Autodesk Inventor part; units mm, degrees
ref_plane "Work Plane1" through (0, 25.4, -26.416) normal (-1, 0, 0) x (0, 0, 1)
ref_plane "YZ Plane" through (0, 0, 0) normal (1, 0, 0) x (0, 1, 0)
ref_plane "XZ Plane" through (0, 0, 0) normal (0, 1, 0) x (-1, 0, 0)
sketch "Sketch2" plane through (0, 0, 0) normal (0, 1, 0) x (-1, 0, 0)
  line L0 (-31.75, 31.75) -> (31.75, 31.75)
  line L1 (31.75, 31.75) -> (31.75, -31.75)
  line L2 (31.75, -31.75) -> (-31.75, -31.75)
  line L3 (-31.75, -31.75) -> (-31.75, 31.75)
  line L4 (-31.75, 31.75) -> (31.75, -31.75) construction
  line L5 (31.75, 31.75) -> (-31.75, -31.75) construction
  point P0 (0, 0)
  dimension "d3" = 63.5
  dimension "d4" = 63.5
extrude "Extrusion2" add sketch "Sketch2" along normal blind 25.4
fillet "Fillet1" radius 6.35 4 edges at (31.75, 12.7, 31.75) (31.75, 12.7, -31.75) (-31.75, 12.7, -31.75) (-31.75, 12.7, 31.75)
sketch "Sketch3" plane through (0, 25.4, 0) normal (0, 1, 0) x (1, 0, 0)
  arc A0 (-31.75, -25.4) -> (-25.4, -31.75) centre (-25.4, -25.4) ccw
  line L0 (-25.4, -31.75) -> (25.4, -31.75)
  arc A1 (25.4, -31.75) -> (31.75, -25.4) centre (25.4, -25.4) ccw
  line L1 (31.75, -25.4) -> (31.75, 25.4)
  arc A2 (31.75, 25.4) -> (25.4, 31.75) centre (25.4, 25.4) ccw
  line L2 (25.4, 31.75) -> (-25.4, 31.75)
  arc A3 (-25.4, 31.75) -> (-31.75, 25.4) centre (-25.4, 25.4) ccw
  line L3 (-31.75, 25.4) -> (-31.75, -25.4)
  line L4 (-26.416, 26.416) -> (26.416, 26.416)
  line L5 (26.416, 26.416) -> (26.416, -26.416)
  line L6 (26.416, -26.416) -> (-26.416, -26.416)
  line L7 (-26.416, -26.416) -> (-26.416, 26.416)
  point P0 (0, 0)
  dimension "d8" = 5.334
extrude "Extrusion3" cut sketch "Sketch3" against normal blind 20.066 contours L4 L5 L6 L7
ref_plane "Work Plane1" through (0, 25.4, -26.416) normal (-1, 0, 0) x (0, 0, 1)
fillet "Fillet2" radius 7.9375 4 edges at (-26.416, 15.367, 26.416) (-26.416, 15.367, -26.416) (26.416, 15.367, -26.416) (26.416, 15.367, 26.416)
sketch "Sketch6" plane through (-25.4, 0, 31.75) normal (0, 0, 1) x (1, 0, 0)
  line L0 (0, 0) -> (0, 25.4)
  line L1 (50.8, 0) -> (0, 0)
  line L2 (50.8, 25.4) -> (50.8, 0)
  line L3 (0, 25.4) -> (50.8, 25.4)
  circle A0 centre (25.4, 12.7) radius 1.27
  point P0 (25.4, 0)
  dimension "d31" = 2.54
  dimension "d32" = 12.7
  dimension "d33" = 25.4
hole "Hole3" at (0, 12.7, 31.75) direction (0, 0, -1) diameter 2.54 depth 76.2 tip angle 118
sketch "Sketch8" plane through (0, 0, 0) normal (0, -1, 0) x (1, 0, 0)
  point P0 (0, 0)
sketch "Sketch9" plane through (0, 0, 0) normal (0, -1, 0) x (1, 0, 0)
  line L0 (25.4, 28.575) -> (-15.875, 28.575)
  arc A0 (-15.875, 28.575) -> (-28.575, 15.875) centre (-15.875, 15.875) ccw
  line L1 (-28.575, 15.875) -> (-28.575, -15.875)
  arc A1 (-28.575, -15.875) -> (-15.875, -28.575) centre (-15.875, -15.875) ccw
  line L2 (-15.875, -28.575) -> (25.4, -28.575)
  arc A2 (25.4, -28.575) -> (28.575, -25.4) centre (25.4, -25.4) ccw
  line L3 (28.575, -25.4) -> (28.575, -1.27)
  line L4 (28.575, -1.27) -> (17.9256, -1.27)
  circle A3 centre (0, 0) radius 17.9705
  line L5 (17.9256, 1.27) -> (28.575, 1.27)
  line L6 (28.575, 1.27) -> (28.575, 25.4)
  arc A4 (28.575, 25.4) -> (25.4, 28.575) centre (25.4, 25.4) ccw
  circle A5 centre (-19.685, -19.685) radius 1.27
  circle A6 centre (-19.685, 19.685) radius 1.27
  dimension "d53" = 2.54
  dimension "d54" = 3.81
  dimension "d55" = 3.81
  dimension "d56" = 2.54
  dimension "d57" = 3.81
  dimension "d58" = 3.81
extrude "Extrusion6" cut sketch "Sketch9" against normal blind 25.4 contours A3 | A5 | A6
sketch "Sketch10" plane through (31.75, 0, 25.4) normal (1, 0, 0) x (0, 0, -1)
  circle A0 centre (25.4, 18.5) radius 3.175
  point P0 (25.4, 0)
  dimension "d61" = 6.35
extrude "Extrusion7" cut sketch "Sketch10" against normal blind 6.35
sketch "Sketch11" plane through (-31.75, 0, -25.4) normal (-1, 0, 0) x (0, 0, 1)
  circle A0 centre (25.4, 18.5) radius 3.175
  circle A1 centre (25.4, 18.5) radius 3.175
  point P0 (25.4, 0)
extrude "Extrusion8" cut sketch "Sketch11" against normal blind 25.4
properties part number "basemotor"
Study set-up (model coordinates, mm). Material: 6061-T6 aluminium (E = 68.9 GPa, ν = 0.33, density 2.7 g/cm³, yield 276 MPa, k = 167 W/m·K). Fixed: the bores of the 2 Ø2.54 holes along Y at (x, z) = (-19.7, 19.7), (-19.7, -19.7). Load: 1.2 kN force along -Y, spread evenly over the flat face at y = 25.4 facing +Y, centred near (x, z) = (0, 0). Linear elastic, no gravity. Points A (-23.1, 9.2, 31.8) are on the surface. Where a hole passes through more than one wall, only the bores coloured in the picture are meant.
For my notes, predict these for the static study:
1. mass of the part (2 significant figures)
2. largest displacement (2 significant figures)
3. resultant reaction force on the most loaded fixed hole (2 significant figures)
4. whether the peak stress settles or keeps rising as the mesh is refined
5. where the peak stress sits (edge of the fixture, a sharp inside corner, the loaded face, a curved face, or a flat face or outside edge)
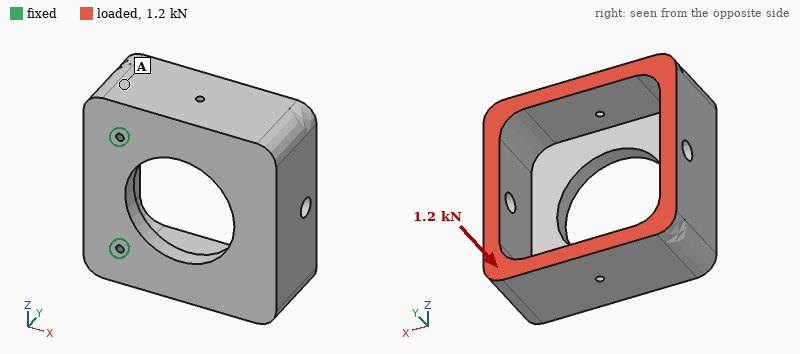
110 g
0.23 mm
630 N
keeps rising
edge of the fixture
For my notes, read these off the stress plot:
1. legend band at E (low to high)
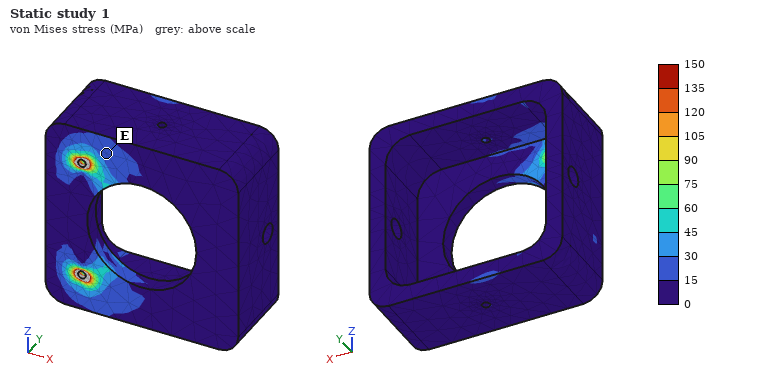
15 to 30 MPa
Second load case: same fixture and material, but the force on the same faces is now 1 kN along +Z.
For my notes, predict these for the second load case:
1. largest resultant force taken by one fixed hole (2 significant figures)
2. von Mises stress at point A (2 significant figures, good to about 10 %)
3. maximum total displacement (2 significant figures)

840 N
8.3 MPa
76 µm
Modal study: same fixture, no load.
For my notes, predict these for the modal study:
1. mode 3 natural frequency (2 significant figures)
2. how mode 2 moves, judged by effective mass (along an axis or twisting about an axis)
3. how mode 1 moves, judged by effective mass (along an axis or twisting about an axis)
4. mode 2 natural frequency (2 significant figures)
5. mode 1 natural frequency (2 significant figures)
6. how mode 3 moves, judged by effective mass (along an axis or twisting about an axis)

3600 Hz
along Z
along Y
2500 Hz
1200 Hz
along Z
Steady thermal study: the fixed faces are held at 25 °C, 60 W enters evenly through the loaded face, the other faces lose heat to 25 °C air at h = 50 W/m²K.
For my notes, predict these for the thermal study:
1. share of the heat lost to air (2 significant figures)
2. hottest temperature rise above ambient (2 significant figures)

22 %
29 K
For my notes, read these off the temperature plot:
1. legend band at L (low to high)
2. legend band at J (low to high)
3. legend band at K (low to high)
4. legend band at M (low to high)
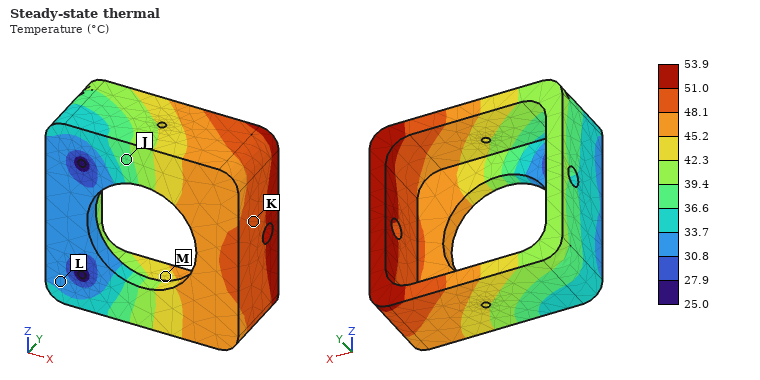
30.8 to 33.7 °C
36.6 to 39.4 °C
48.1 to 51.0 °C
42.3 to 45.2 °C
